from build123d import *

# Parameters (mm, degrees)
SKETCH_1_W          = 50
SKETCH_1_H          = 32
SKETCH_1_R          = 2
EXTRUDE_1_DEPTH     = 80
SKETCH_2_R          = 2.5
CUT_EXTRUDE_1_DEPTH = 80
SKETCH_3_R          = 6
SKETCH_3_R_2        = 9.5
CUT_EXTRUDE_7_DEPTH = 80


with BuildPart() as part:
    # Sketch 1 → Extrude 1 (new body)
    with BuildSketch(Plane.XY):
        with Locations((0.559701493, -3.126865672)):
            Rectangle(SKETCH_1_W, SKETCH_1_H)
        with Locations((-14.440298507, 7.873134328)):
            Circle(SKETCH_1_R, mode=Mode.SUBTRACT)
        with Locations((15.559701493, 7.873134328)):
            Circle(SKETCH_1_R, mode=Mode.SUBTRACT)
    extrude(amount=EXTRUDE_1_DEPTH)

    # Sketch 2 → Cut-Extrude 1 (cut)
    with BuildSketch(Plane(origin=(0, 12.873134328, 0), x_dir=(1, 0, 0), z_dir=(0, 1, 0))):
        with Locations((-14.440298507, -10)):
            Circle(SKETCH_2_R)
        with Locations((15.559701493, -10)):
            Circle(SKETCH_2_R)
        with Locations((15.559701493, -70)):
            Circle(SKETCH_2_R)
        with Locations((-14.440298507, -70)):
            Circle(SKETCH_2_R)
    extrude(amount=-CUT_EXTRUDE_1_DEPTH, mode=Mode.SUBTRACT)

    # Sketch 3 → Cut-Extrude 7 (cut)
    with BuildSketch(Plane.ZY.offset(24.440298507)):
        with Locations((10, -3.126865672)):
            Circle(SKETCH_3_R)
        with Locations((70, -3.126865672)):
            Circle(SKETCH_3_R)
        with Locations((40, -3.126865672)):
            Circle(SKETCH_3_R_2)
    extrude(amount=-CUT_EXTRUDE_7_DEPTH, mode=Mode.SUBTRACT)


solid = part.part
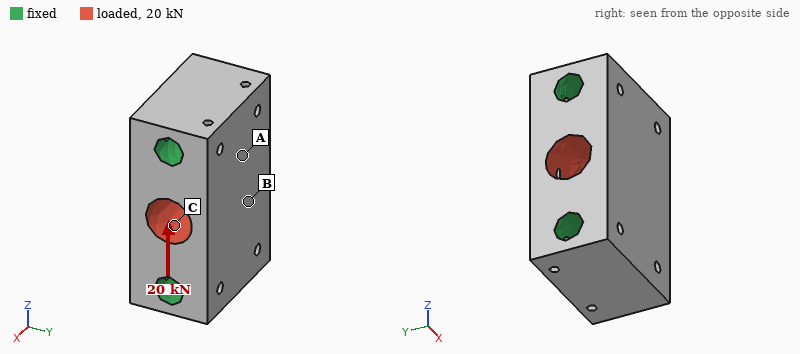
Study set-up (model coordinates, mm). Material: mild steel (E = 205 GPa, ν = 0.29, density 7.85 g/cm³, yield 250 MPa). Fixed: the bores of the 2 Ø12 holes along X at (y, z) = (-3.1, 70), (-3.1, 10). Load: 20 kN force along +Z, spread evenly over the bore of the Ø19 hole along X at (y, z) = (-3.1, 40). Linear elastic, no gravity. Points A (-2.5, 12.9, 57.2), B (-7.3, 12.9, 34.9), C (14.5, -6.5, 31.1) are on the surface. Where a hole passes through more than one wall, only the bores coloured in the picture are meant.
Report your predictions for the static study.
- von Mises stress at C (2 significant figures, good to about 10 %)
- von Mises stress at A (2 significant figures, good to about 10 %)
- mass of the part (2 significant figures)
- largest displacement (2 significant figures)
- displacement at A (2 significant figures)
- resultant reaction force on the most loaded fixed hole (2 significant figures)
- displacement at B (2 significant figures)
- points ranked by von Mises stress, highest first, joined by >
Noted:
9.5 MPa
3.4 MPa
780 g
1.1 µm
0.55 µm
10 kN
0.66 µm
C > A > B
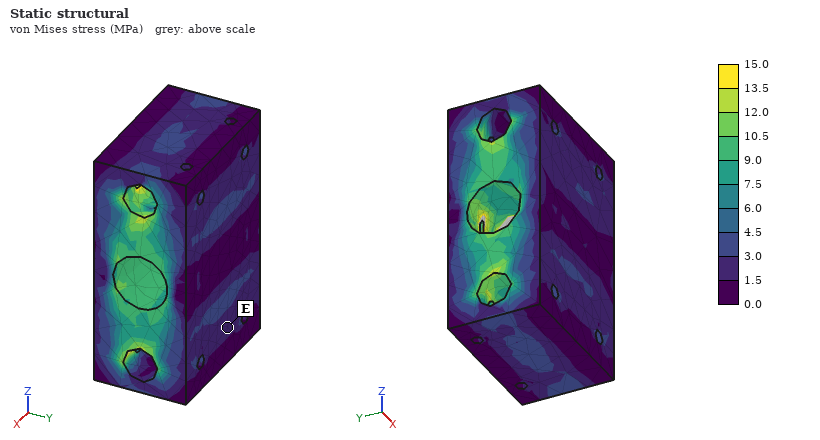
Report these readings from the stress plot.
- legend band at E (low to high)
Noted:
1.5 to 3.0 MPa
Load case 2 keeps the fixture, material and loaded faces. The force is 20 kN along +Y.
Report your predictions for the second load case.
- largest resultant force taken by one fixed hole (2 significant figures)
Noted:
10 kN
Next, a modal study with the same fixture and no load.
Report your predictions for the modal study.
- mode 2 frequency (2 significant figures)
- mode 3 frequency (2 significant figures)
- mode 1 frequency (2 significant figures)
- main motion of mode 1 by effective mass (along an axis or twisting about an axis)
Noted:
28 kHz
29 kHz
25 kHz
along Y
